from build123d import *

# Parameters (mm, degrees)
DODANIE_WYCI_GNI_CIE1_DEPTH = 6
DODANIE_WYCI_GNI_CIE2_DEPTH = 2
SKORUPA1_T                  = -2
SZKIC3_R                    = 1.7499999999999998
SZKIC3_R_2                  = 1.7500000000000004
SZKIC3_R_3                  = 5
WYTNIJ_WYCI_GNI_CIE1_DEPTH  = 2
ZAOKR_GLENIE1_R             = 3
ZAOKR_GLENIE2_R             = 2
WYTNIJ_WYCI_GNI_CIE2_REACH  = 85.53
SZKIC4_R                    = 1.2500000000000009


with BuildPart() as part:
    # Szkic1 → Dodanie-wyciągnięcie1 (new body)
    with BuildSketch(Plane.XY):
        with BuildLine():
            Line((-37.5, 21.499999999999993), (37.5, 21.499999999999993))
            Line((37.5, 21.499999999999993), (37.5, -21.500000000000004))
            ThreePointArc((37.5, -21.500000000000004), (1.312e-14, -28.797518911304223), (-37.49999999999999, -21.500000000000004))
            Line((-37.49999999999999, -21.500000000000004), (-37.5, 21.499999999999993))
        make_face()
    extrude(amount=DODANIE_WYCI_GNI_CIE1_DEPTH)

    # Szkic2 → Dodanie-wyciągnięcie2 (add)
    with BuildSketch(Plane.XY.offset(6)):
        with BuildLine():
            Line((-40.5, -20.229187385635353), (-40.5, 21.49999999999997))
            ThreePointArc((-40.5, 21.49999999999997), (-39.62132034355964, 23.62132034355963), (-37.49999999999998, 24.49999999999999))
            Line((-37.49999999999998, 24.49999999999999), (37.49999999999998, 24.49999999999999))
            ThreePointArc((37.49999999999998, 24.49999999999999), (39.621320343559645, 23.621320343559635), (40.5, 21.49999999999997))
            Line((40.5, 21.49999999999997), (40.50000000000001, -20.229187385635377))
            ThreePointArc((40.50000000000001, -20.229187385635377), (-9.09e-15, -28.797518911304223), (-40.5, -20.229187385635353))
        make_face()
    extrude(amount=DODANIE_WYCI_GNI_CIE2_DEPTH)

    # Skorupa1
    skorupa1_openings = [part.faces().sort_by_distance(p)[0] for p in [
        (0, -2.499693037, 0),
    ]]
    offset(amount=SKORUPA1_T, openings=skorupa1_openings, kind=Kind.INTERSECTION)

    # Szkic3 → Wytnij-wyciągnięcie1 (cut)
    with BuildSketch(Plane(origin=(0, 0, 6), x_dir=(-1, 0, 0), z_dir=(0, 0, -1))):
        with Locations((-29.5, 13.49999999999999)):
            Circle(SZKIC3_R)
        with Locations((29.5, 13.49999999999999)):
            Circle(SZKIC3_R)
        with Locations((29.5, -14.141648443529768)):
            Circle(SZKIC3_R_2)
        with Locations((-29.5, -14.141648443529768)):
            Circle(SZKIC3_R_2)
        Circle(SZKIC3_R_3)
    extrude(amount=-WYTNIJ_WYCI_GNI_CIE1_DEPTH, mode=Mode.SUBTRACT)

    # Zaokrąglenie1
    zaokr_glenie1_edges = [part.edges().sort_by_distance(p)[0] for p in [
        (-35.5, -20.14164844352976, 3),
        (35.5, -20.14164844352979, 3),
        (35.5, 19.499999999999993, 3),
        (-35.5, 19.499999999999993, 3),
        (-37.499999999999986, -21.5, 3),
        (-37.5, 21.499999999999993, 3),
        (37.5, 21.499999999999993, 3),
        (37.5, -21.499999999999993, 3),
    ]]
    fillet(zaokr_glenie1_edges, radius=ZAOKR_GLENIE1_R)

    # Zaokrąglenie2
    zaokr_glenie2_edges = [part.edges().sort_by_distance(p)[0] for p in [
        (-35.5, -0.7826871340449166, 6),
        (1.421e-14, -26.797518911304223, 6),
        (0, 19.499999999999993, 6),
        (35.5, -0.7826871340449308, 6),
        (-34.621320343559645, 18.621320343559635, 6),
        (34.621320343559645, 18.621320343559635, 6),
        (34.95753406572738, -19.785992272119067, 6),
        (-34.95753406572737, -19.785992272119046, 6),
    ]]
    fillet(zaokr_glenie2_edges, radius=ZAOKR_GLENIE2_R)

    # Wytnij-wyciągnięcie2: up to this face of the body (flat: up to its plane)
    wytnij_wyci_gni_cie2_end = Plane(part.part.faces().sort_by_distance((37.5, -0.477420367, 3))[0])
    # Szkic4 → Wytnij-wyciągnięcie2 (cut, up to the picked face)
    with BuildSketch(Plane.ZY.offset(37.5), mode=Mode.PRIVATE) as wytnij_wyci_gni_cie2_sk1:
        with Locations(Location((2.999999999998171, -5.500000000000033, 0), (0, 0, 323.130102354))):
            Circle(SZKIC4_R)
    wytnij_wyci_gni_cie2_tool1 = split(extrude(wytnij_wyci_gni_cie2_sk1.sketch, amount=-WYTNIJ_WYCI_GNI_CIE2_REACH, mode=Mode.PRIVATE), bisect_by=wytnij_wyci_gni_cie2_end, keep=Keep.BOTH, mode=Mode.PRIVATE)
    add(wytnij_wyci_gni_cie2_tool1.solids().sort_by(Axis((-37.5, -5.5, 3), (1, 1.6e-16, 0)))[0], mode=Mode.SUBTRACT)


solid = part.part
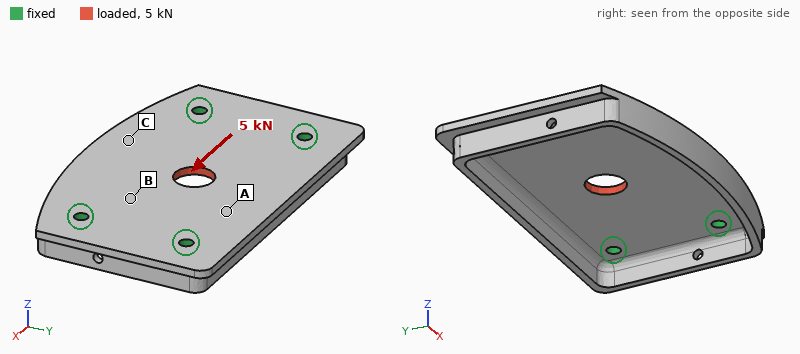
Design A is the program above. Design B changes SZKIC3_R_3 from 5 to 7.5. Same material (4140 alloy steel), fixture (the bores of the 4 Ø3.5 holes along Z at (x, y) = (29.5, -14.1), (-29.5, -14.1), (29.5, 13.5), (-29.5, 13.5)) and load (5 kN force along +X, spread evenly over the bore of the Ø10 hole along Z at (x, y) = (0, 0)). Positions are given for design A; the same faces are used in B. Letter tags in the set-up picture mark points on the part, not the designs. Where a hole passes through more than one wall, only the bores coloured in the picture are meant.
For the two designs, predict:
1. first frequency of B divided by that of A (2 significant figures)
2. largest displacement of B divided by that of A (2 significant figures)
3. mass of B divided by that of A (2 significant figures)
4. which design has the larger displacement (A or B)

1.0
0.83
0.98
A
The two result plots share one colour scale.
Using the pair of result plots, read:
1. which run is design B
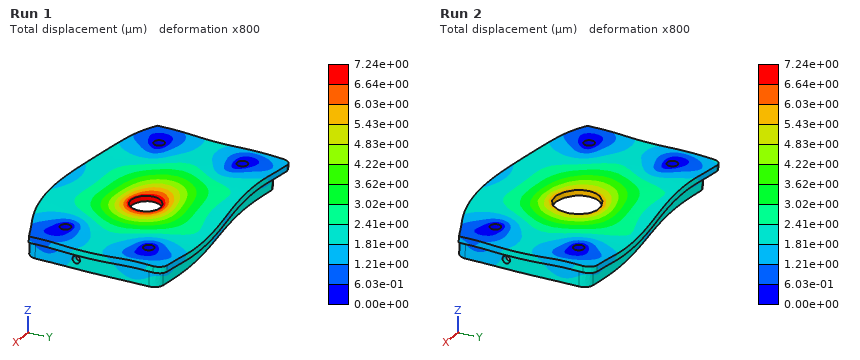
Run 2
